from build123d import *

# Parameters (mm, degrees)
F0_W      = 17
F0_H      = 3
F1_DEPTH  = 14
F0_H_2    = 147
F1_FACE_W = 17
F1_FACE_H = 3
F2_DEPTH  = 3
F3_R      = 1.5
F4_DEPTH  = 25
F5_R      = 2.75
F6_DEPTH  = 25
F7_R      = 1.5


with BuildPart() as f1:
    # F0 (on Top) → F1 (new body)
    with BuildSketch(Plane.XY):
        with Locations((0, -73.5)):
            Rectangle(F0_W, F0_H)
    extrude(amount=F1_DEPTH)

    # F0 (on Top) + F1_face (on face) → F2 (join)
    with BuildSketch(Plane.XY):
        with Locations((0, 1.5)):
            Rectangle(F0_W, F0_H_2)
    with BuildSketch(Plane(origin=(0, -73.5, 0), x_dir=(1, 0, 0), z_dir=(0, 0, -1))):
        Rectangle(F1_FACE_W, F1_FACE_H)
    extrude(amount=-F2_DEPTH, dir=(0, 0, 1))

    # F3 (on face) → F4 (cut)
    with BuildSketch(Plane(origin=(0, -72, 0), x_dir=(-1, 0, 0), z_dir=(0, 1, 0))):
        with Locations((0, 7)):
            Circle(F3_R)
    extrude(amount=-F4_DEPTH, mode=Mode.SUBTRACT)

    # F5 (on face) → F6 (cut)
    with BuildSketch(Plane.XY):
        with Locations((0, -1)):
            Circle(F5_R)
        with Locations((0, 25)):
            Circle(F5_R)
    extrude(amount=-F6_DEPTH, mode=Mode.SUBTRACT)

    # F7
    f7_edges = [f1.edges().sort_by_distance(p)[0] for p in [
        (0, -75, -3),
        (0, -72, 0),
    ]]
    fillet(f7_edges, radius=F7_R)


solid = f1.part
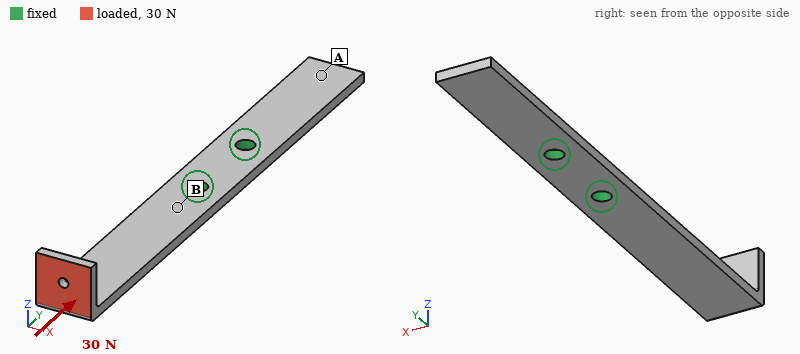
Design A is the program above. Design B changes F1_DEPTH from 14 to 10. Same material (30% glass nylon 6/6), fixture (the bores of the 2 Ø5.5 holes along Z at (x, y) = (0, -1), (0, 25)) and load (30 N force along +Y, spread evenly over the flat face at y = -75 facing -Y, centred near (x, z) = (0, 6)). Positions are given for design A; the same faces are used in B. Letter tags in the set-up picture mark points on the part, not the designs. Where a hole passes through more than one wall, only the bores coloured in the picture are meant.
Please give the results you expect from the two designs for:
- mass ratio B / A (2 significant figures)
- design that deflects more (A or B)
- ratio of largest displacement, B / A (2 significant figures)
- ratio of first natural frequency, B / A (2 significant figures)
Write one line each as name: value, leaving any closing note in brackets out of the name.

mass ratio B / A: 0.98
design that deflects more: A
ratio of largest displacement, B / A: 0.70
ratio of first natural frequency, B / A: 1.1
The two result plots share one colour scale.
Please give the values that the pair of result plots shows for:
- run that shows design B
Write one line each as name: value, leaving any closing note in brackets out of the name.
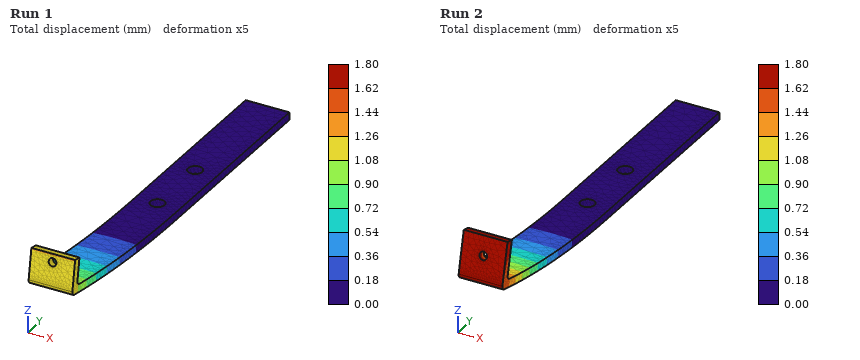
run that shows design B: Run 1
